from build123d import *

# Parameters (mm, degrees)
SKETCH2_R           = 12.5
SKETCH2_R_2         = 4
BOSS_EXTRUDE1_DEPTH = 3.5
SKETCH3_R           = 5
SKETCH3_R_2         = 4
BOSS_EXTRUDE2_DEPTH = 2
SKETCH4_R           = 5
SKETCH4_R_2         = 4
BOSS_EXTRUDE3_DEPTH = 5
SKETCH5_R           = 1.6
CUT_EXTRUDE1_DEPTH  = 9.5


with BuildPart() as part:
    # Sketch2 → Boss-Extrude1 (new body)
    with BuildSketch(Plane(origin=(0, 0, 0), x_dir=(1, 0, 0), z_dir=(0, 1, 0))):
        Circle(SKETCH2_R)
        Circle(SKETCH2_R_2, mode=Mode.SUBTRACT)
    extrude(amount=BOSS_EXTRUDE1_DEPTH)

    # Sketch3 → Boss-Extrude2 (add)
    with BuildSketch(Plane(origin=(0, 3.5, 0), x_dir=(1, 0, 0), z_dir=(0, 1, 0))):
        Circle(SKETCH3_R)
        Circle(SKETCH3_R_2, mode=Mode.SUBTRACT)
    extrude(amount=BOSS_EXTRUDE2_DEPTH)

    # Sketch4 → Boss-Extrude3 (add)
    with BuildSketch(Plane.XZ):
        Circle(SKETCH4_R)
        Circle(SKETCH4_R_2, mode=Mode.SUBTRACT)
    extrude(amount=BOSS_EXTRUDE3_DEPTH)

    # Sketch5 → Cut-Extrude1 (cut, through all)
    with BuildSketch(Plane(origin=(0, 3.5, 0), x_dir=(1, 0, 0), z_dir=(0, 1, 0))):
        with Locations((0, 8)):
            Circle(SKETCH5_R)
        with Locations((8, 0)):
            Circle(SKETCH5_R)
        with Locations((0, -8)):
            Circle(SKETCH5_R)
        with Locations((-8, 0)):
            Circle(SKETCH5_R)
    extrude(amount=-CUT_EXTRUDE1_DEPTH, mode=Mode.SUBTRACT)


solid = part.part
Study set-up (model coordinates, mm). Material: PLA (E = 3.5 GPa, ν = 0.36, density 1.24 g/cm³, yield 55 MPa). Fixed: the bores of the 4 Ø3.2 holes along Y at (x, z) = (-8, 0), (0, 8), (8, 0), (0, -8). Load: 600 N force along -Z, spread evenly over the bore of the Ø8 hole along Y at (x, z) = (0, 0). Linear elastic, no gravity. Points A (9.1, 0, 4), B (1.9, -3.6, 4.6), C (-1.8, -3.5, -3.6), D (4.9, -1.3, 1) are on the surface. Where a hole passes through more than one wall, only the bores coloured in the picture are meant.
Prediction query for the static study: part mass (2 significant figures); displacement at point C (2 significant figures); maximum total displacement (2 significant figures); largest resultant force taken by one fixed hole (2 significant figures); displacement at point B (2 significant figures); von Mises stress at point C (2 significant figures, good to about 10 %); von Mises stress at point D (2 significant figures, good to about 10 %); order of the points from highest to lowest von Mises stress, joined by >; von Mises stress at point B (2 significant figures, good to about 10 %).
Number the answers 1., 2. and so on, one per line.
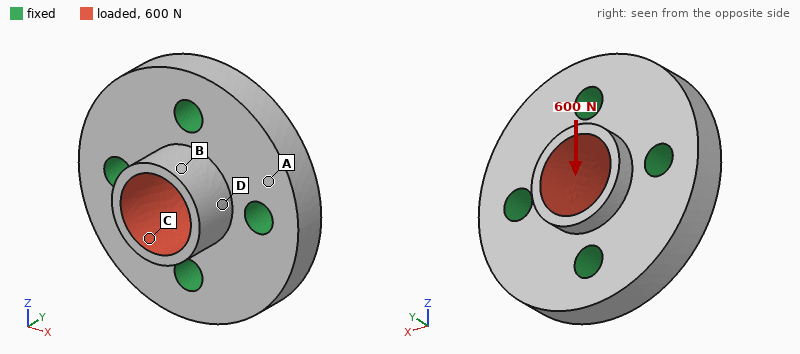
1. 2.0 g
2. 61 µm
3. 79 µm
4. 180 N
5. 63 µm
6. 13 MPa
7. 17 MPa
8. D > C > B > A
9. 9.0 MPa
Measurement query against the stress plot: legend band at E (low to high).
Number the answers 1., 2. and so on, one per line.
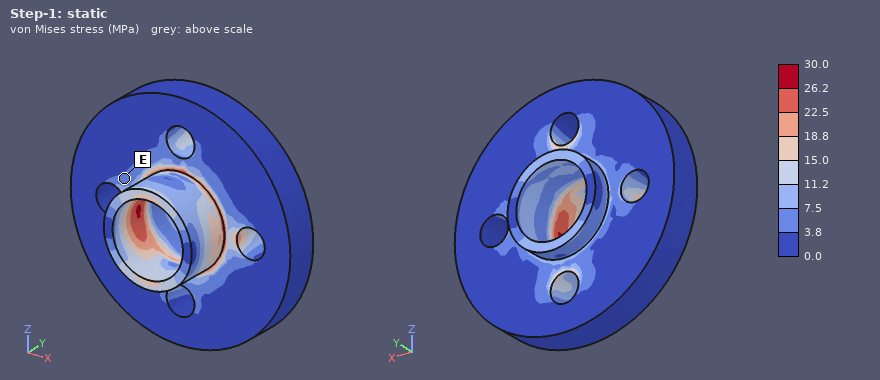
1. 3.8 to 7.5 MPa
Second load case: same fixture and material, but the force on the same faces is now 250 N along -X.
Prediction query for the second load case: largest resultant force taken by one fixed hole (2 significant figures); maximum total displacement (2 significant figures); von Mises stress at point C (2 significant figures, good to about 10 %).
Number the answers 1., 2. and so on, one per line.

1. 76 N
2. 33 µm
3. 6.0 MPa
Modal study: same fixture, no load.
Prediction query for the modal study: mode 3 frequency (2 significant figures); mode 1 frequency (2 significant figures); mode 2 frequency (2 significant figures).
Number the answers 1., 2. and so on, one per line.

1. 23 kHz
2. 21 kHz
3. 22 kHz
